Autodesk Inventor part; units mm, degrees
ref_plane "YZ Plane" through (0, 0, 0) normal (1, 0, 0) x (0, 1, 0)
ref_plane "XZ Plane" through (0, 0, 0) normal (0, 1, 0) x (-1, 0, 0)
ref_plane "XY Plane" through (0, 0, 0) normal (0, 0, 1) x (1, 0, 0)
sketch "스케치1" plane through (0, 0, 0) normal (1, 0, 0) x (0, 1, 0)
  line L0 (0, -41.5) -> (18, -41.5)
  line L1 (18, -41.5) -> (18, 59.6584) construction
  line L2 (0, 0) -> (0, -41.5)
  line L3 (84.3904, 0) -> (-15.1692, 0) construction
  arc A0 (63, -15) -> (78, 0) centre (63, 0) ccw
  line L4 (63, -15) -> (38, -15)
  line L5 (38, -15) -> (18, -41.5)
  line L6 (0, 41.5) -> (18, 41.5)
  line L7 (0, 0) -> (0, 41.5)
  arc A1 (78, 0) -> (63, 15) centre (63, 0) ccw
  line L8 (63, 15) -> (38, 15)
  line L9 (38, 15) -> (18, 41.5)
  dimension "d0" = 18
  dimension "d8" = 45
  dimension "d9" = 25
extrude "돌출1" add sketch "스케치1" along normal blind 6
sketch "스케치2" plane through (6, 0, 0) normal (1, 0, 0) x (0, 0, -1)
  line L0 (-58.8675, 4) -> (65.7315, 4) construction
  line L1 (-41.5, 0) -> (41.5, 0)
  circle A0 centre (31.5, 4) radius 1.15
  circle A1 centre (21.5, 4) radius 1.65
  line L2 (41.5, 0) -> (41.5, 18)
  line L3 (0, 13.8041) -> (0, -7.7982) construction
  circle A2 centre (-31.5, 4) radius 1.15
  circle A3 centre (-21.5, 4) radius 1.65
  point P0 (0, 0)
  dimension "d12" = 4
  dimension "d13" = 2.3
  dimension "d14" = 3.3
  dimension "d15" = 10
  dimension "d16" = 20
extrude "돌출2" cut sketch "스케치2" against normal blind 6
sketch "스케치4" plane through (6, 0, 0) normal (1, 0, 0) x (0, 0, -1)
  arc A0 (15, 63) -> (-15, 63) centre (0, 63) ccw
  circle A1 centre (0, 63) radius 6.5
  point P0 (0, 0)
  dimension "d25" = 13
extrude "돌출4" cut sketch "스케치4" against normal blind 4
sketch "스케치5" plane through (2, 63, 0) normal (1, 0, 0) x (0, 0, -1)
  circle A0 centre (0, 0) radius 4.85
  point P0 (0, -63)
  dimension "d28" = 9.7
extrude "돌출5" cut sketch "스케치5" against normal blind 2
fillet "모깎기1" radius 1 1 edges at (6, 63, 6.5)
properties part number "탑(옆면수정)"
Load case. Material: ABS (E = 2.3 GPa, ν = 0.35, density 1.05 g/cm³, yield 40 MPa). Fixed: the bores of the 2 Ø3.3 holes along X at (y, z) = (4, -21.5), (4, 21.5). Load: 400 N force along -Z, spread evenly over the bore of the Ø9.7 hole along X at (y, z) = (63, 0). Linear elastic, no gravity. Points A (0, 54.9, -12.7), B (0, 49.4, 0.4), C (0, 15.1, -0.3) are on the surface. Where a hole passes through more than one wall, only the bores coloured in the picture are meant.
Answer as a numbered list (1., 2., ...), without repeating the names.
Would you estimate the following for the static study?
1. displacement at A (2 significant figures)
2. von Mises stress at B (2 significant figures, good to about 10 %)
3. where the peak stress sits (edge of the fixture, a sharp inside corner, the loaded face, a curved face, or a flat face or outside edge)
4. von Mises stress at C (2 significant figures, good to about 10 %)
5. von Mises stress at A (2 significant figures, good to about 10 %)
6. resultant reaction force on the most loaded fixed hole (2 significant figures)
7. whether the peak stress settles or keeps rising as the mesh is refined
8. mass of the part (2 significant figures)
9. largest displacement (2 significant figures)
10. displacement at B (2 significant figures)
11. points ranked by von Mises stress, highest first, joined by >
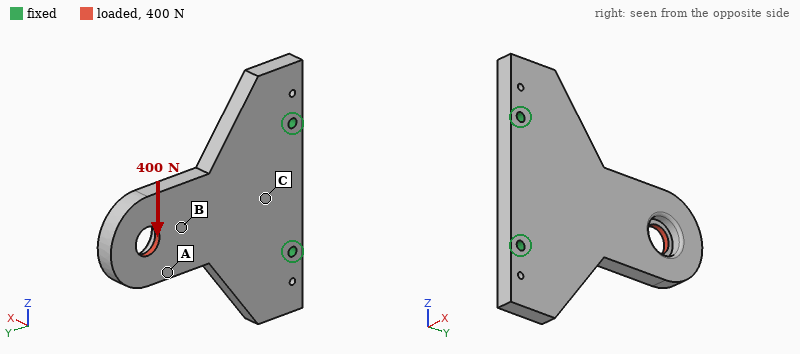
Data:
1. 0.41 mm
2. 11 MPa
3. edge of the fixture
4. 2.3 MPa
5. 6.7 MPa
6. 570 N
7. keeps rising
8. 23 g
9. 0.65 mm
10. 0.27 mm
11. B > A > C
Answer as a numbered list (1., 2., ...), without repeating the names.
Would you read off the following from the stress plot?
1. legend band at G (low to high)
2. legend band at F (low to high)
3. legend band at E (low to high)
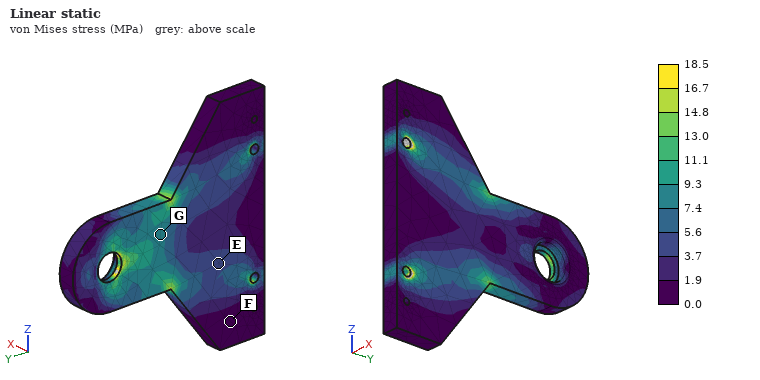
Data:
1. 7.4 to 9.3 MPa
2. 0.0 to 1.9 MPa
3. 3.7 to 5.6 MPa
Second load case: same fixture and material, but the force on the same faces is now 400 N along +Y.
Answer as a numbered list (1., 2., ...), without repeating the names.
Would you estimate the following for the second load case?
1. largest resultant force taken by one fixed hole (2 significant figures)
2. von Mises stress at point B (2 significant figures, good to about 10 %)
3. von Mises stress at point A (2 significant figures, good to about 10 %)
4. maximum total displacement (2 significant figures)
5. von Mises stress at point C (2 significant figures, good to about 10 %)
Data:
1. 210 N
2. 6.5 MPa
3. 5.9 MPa
4. 1.3 mm
5. 2.3 MPa
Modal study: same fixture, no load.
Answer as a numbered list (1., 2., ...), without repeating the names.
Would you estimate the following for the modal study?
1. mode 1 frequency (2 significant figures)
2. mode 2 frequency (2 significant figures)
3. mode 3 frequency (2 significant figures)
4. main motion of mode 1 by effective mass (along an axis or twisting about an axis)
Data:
1. 350 Hz
2. 1500 Hz
3. 1500 Hz
4. along X
